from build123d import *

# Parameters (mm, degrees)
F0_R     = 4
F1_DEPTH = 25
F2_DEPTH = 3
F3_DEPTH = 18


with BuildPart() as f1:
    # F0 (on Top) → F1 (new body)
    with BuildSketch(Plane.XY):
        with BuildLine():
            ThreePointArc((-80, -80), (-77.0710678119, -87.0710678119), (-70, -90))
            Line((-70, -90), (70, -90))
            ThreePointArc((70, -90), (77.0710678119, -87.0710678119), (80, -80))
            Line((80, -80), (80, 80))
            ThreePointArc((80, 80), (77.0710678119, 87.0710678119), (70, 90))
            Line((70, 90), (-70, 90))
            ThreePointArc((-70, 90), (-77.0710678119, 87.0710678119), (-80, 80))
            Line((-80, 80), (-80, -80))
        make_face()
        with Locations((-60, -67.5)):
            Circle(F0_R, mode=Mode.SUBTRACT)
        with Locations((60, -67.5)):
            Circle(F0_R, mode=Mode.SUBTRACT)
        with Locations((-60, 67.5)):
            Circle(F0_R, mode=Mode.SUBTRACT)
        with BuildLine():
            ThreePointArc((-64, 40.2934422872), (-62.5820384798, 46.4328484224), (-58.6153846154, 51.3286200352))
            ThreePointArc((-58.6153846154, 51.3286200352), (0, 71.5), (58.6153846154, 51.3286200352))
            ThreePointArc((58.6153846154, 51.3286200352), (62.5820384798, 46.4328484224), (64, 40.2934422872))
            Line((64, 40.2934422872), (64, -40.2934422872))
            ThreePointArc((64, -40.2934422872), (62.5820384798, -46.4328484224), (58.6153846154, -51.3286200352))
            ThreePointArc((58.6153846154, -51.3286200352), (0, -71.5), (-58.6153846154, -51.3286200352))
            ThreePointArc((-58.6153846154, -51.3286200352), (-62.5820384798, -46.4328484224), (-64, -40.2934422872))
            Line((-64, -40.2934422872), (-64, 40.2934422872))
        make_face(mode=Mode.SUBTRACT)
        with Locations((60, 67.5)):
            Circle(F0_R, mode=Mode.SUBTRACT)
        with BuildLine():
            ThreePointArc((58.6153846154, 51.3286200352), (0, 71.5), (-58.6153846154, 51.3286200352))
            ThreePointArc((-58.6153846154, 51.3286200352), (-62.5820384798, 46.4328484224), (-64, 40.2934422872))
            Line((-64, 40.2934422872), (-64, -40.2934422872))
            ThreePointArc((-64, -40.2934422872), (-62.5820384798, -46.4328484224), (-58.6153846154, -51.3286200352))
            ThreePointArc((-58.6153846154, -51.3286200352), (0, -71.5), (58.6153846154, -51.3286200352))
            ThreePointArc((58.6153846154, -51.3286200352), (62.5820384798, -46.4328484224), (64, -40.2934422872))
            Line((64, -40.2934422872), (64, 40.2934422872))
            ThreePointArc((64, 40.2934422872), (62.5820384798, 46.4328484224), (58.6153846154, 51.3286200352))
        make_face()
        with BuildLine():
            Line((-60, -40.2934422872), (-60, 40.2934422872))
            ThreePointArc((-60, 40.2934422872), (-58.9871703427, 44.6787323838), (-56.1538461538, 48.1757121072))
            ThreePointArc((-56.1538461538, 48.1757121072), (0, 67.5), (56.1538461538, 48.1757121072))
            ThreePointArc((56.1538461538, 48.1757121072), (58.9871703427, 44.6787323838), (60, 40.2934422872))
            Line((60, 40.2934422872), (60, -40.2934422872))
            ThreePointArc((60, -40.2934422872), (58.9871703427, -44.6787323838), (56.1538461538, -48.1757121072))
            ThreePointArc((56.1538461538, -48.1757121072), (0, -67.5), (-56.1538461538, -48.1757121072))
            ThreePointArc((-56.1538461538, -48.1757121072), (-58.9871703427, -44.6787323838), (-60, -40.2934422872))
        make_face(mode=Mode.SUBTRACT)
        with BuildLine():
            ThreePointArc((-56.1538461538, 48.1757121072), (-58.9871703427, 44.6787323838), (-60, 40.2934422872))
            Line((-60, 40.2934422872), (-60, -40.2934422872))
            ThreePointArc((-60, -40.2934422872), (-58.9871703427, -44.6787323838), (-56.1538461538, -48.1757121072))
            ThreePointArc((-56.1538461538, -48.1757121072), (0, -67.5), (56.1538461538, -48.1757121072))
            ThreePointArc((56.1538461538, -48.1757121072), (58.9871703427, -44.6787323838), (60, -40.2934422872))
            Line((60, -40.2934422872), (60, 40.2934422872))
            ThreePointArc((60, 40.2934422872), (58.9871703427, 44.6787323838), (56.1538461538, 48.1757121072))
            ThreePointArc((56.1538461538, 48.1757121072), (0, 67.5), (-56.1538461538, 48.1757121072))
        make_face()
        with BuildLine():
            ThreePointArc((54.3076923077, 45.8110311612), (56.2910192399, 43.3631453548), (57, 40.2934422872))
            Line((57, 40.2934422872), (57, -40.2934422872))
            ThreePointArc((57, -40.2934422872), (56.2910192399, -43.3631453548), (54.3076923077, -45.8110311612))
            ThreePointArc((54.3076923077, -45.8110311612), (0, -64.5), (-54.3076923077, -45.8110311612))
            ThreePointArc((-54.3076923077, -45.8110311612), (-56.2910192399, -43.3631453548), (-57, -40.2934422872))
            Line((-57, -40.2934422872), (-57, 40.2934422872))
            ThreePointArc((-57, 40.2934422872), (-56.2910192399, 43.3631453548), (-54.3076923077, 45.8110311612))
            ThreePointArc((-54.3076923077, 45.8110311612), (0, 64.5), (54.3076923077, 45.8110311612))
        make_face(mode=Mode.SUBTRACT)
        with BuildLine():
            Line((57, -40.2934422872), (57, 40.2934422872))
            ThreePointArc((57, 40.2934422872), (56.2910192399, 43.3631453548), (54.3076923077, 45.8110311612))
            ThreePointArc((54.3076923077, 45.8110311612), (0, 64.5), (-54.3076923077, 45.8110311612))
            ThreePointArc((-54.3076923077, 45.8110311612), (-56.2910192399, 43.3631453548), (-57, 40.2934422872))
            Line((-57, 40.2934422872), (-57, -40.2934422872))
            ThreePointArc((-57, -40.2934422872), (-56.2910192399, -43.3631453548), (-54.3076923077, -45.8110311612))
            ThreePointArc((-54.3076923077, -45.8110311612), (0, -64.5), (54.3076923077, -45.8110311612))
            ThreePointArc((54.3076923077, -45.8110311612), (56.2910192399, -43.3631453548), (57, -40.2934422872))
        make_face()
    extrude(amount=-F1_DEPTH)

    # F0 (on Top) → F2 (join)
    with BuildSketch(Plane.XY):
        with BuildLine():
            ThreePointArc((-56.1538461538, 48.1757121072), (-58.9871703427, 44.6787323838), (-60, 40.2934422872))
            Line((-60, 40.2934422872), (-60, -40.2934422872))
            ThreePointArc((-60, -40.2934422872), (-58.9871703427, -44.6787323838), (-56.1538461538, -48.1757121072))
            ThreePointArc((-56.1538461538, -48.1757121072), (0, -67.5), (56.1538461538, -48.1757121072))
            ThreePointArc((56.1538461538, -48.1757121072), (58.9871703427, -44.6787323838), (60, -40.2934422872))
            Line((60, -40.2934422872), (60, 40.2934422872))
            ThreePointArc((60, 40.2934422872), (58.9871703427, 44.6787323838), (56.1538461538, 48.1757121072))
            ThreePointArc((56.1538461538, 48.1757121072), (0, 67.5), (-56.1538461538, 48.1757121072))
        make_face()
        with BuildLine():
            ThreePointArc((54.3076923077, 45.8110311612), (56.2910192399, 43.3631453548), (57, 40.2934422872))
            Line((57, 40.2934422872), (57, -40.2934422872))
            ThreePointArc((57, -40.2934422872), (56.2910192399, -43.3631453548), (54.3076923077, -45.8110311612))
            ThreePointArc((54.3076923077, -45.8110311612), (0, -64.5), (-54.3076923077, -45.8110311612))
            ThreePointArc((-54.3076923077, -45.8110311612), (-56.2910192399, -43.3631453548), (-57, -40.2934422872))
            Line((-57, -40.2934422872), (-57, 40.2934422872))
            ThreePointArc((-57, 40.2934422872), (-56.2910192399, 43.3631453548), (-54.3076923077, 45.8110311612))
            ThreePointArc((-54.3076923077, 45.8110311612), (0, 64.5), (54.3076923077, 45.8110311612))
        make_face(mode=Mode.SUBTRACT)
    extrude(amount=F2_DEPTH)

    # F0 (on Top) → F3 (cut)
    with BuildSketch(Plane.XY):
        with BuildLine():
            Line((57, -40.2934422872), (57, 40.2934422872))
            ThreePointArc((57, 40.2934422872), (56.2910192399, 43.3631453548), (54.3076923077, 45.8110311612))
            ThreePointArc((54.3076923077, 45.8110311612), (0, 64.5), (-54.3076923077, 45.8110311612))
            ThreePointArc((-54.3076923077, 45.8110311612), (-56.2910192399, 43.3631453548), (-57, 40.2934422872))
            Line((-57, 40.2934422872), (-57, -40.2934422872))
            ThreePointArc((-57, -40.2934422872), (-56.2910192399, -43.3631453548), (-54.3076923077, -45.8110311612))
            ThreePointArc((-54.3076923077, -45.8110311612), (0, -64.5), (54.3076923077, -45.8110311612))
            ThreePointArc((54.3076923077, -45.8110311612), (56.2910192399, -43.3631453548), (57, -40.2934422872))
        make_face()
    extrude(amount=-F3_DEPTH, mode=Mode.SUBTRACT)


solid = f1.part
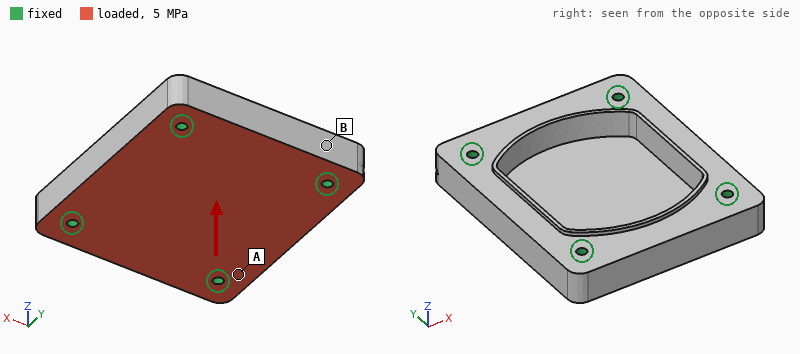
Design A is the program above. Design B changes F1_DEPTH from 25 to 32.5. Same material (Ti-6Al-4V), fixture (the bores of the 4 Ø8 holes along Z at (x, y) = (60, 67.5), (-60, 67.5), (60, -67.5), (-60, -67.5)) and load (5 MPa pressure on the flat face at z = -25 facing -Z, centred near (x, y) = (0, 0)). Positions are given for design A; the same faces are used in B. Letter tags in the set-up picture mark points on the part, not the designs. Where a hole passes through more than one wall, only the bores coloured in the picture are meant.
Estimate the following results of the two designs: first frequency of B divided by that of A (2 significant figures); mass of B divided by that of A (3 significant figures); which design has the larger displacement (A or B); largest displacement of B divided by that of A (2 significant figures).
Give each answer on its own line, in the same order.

1.4
1.45
A
0.22
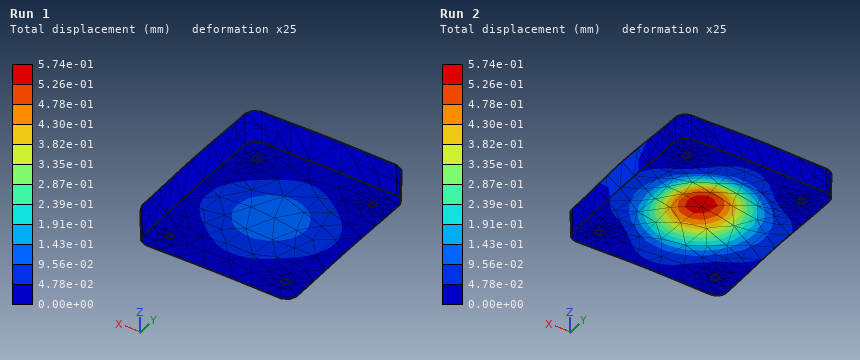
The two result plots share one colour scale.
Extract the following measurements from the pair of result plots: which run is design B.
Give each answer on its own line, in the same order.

Run 1
